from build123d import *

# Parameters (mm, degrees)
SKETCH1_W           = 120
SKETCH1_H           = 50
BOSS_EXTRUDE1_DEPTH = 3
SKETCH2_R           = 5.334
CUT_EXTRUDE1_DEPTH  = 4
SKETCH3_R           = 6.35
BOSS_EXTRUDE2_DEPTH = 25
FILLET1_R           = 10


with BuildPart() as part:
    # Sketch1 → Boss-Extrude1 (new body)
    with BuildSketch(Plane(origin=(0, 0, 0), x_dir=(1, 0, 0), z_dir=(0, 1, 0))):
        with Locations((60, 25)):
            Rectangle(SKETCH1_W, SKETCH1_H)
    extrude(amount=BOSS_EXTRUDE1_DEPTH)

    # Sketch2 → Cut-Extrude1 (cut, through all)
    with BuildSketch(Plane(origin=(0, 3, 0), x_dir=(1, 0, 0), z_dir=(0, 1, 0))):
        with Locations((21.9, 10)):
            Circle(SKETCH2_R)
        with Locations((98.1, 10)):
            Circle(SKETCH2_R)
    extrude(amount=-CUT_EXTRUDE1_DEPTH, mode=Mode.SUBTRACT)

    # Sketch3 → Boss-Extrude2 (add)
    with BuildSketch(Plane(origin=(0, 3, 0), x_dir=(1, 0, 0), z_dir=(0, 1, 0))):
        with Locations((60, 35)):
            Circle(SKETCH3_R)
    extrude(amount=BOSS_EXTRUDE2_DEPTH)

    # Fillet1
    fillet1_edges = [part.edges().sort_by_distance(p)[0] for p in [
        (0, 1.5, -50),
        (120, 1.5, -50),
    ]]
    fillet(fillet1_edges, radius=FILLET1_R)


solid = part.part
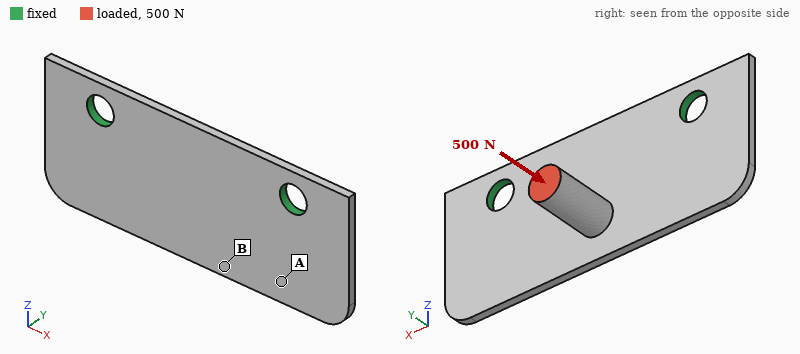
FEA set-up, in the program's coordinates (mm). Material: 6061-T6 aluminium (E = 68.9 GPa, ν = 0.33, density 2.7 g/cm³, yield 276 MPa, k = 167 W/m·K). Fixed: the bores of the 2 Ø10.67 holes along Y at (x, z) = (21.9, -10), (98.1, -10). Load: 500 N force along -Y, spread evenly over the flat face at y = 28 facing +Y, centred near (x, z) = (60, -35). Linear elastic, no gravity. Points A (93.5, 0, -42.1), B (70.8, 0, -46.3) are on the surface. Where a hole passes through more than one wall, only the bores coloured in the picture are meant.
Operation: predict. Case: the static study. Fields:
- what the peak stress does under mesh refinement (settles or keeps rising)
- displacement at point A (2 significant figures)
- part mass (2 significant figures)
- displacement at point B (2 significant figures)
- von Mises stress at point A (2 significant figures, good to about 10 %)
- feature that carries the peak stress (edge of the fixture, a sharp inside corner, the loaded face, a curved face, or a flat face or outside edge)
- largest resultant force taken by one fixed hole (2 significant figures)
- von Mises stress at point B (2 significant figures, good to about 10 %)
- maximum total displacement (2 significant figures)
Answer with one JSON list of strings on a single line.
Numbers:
["keeps rising", "0.23 mm", "55 g", "0.46 mm", "25 MPa", "edge of the fixture", "250 N", "52 MPa", "0.54 mm"]
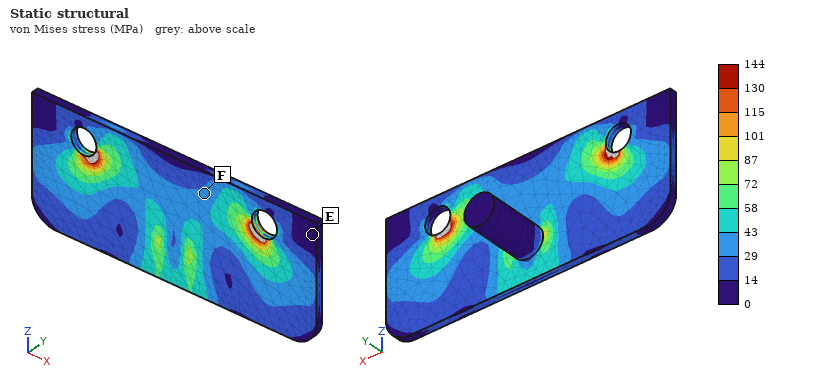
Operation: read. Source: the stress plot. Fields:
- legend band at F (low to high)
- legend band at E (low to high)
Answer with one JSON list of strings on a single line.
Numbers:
["29 to 43 MPa", "0 to 14 MPa"]
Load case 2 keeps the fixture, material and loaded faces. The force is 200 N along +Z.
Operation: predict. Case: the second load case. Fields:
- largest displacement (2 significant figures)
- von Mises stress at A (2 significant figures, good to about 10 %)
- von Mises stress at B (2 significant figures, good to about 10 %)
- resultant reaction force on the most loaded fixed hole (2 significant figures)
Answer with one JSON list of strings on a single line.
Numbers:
["0.37 mm", "18 MPa", "25 MPa", "110 N"]
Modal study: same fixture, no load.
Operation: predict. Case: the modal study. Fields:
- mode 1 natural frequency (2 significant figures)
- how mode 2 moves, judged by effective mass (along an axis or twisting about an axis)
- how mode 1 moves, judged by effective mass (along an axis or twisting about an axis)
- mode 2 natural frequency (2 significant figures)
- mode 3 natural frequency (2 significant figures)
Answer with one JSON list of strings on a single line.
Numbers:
["1100 Hz", "twisting about Z", "along Y", "2100 Hz", "2500 Hz"]
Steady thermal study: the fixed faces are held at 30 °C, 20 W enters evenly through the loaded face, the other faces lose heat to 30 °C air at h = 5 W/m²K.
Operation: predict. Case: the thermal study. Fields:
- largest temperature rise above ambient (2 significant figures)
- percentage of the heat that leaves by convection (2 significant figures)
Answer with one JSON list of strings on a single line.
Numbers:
["47 K", "3.4 %"]
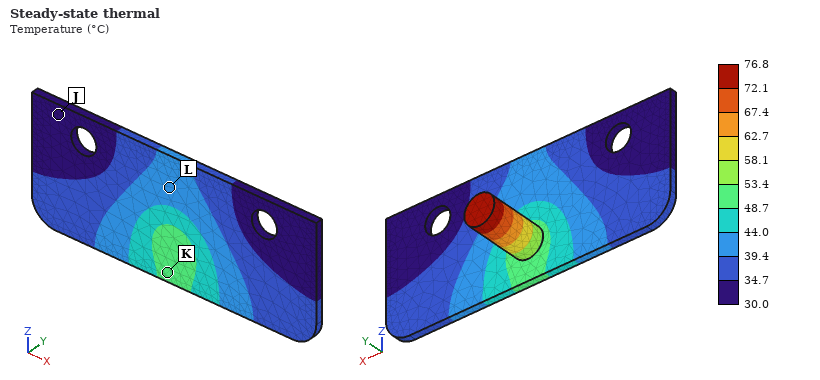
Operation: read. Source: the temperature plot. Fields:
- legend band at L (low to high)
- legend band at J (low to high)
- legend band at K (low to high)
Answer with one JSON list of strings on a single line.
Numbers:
["39.4 to 44.0 °C", "30.0 to 34.7 °C", "48.7 to 53.4 °C"]
